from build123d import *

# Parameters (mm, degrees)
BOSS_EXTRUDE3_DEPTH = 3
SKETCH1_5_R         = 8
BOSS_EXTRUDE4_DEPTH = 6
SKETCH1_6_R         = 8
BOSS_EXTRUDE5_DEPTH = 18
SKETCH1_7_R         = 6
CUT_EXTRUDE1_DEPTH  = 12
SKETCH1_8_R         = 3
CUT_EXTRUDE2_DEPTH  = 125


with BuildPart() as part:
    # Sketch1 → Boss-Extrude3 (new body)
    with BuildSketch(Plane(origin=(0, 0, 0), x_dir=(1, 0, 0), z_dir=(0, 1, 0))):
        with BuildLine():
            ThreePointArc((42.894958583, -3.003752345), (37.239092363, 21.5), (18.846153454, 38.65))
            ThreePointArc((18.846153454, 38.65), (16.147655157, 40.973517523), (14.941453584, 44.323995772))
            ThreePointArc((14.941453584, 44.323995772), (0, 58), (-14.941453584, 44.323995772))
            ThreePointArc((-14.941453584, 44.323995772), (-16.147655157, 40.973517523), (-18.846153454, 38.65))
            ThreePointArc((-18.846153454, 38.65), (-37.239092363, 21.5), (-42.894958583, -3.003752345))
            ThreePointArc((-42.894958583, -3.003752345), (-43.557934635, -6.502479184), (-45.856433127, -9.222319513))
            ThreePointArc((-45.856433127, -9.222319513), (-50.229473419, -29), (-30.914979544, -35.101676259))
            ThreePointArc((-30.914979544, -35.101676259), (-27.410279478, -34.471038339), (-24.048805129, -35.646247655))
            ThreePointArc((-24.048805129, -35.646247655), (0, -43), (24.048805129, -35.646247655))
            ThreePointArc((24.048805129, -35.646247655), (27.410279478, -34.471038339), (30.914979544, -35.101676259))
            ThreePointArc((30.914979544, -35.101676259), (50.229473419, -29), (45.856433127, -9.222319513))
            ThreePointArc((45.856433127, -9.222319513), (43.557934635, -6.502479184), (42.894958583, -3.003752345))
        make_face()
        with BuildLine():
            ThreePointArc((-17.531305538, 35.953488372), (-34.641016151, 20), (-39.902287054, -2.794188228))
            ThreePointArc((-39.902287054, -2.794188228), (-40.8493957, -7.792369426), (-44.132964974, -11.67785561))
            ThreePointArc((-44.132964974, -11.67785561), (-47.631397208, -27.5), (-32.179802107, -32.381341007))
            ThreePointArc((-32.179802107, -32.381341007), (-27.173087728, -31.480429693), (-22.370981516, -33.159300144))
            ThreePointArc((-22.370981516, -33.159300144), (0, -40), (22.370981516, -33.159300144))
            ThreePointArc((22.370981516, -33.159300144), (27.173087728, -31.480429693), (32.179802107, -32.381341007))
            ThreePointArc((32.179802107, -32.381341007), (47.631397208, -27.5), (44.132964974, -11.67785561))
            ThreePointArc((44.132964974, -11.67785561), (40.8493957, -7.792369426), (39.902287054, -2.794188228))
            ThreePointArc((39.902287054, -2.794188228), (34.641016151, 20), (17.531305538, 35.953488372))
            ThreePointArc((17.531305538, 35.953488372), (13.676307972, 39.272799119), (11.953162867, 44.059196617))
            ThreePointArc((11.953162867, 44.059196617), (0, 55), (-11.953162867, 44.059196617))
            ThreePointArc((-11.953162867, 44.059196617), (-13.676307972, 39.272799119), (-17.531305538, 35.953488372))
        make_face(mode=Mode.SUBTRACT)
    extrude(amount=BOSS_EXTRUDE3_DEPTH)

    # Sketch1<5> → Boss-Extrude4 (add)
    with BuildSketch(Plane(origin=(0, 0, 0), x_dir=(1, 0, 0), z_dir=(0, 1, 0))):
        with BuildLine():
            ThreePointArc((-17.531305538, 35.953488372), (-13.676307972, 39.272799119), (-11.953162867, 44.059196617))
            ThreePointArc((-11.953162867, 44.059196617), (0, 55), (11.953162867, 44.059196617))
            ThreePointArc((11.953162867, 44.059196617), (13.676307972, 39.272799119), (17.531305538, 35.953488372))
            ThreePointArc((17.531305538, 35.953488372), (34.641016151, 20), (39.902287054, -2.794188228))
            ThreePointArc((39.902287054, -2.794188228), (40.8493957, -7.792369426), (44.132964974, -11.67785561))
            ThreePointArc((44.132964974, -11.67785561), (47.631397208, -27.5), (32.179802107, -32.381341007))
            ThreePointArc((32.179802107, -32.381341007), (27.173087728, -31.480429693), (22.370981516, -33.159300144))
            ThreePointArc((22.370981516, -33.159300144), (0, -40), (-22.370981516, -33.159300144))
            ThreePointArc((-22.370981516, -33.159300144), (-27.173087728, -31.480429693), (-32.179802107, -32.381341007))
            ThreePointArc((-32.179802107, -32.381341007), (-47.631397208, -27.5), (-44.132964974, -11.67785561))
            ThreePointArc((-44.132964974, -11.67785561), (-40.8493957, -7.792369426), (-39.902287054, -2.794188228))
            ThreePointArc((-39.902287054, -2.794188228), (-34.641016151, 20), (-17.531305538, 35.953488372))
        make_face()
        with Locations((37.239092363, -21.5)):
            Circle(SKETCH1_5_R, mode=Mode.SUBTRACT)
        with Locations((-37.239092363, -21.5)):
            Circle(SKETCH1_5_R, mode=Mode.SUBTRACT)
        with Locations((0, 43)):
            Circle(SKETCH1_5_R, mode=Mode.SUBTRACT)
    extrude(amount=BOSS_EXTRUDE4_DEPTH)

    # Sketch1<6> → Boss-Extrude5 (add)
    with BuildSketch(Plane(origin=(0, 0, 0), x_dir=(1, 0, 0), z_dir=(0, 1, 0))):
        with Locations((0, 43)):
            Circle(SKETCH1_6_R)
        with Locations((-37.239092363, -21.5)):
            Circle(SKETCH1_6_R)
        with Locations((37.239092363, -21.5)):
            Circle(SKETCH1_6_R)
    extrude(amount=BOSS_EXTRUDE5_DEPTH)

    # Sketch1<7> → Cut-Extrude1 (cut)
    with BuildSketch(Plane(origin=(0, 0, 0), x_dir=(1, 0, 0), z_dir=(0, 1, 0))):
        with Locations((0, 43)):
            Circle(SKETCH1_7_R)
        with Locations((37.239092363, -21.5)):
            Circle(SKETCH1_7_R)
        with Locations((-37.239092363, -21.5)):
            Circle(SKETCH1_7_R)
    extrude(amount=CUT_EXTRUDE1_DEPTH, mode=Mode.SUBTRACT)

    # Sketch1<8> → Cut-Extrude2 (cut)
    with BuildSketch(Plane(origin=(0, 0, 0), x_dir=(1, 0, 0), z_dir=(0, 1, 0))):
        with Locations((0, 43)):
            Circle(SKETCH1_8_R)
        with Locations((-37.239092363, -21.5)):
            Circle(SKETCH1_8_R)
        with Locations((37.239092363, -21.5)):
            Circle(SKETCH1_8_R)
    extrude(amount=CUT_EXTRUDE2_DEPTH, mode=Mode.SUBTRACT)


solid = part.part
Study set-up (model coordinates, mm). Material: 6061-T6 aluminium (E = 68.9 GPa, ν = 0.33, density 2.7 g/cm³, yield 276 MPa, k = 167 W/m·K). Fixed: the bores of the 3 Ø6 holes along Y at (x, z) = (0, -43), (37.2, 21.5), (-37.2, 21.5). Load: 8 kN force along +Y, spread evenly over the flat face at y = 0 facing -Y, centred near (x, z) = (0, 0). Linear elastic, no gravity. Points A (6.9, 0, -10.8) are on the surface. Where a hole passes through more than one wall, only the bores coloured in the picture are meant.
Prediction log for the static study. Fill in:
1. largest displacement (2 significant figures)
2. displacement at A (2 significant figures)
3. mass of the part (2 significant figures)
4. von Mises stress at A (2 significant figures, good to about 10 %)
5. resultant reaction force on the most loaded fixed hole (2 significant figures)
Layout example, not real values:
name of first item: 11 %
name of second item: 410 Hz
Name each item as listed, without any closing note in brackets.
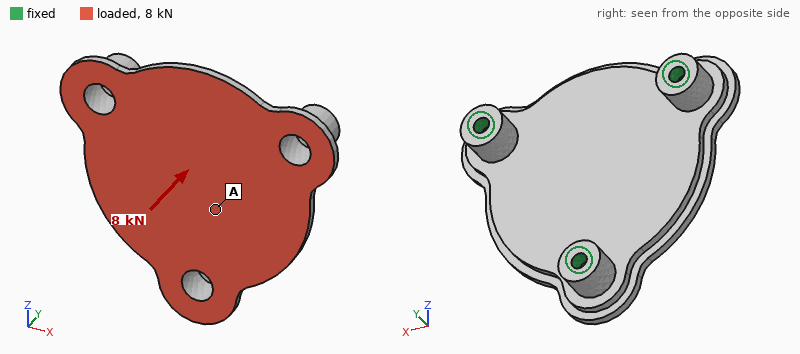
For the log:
largest displacement: 0.12 mm
displacement at A: 0.11 mm
mass of the part: 110 g
von Mises stress at A: 43 MPa
resultant reaction force on the most loaded fixed hole: 3.0 kN
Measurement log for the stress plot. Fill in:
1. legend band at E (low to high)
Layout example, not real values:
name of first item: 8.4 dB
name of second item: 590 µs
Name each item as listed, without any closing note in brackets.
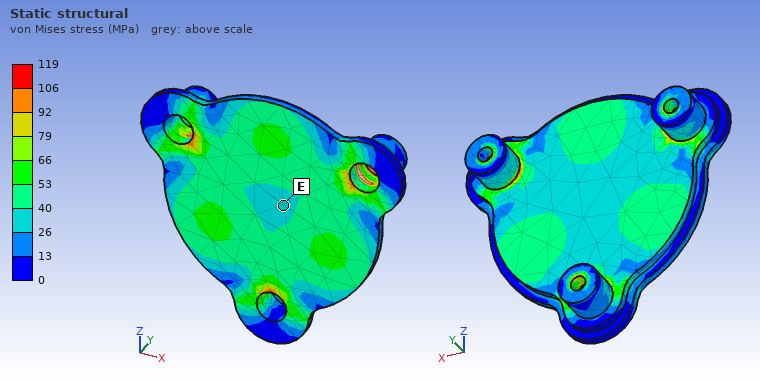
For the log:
legend band at E: 26 to 40 MPa
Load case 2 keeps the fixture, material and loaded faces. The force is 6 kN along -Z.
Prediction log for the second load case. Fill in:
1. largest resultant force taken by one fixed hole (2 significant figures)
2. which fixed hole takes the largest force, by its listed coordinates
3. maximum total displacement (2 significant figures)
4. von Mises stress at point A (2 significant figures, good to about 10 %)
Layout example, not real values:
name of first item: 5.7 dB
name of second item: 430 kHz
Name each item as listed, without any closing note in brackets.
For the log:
largest resultant force taken by one fixed hole: 2.3 kN
which fixed hole takes the largest force, by its listed coordinates: (0, -43)
maximum total displacement: 64 µm
von Mises stress at point A: 17 MPa
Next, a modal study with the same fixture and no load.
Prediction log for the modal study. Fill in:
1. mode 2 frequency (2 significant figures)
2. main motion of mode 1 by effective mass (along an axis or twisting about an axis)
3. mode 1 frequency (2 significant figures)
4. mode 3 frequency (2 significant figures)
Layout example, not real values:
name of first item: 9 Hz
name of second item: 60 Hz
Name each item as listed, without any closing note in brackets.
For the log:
mode 2 frequency: 4900 Hz
main motion of mode 1 by effective mass: along Y
mode 1 frequency: 4600 Hz
mode 3 frequency: 4900 Hz
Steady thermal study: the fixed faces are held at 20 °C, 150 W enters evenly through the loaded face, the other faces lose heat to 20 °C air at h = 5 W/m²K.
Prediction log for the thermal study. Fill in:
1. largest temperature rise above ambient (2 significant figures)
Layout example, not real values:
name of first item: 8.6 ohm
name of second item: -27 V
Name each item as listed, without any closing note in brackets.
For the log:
largest temperature rise above ambient: 57 K
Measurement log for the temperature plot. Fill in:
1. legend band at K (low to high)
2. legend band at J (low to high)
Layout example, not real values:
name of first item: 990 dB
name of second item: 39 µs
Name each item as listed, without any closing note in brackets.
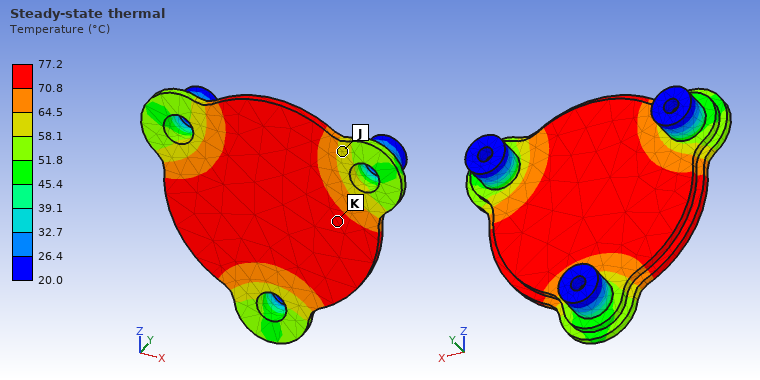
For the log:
legend band at K: 70.8 to 77.2 °C
legend band at J: 58.1 to 64.5 °C
